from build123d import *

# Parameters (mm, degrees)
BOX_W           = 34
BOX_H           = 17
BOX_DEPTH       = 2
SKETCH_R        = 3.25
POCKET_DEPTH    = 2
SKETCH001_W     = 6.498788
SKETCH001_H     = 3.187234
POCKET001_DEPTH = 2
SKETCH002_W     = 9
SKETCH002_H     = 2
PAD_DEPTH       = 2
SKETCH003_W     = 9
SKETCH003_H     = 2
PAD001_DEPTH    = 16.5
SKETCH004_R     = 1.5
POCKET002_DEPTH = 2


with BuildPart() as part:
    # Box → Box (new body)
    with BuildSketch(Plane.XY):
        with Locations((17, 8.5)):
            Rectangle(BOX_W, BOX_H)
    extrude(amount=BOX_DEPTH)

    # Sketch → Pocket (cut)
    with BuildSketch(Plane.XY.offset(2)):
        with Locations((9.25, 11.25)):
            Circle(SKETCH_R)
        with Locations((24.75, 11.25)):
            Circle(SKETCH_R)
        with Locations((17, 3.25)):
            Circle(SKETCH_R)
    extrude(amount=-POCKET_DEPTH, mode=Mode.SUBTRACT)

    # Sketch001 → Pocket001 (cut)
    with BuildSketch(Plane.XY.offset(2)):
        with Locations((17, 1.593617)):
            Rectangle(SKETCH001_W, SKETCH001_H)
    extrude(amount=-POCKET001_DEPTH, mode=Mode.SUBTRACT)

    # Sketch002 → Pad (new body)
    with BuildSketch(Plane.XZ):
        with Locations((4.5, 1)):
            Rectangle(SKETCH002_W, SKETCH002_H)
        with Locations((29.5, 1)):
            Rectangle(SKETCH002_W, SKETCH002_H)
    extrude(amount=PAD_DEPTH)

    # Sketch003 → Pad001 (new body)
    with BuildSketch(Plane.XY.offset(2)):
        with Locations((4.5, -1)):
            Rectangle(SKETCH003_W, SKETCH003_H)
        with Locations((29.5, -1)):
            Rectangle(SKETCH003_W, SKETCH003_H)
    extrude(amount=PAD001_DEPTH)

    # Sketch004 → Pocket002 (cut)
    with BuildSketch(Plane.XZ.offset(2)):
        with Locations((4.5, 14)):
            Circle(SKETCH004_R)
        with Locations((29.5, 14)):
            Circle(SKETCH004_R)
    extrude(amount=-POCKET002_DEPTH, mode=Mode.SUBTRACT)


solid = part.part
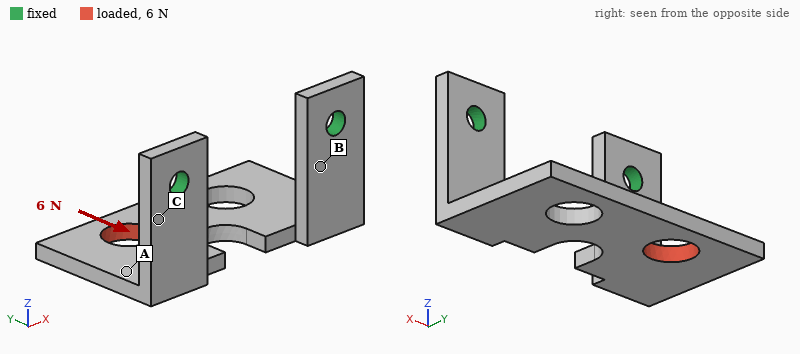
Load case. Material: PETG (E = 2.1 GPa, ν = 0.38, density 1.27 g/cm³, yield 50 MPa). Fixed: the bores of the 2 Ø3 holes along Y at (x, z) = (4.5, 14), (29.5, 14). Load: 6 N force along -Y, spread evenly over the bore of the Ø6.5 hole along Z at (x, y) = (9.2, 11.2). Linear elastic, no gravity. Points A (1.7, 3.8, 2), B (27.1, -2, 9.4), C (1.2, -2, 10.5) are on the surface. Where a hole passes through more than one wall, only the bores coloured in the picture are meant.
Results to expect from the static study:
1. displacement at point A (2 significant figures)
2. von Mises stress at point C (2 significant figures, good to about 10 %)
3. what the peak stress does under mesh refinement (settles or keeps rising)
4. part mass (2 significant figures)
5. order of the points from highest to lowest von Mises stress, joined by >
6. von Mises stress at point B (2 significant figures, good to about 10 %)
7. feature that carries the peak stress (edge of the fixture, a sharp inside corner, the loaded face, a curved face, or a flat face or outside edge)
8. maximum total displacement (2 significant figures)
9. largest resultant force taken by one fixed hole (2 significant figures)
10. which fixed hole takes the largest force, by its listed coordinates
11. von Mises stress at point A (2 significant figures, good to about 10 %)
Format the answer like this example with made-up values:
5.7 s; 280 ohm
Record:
0.20 mm; 5.7 MPa; keeps rising; 2.0 g; C > B > A; 2.8 MPa; edge of the fixture; 0.42 mm; 4.5 N; (4.5, 14); 0.94 MPa
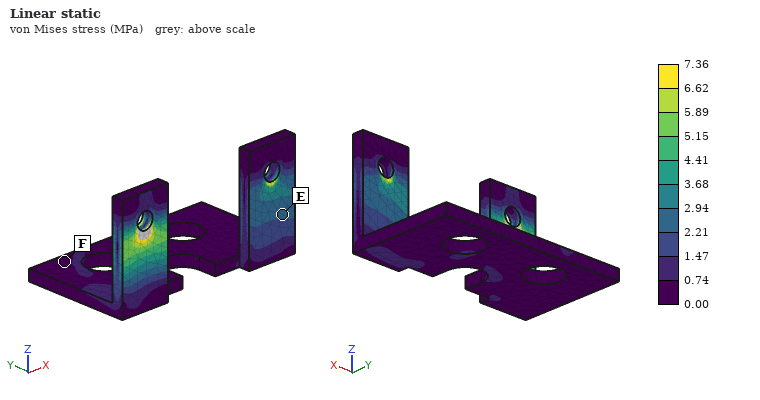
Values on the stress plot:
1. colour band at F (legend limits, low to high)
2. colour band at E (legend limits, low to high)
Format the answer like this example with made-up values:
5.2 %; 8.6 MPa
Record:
0.00 to 0.74 MPa; 2.21 to 2.94 MPa
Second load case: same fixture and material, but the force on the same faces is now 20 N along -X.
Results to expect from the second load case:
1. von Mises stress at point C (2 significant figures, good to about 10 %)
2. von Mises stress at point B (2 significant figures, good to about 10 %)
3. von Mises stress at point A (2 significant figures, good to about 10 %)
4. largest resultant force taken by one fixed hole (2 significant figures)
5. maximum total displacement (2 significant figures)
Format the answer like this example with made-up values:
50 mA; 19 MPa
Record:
9.6 MPa; 4.8 MPa; 4.2 MPa; 13 N; 0.51 mm
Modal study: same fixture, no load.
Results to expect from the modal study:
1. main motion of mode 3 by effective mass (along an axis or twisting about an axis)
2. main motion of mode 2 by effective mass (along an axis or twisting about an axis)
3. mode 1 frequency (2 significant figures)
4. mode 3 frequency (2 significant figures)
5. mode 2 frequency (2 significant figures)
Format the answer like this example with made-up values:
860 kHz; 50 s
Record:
along Y; along X; 490 Hz; 1500 Hz; 960 Hz
